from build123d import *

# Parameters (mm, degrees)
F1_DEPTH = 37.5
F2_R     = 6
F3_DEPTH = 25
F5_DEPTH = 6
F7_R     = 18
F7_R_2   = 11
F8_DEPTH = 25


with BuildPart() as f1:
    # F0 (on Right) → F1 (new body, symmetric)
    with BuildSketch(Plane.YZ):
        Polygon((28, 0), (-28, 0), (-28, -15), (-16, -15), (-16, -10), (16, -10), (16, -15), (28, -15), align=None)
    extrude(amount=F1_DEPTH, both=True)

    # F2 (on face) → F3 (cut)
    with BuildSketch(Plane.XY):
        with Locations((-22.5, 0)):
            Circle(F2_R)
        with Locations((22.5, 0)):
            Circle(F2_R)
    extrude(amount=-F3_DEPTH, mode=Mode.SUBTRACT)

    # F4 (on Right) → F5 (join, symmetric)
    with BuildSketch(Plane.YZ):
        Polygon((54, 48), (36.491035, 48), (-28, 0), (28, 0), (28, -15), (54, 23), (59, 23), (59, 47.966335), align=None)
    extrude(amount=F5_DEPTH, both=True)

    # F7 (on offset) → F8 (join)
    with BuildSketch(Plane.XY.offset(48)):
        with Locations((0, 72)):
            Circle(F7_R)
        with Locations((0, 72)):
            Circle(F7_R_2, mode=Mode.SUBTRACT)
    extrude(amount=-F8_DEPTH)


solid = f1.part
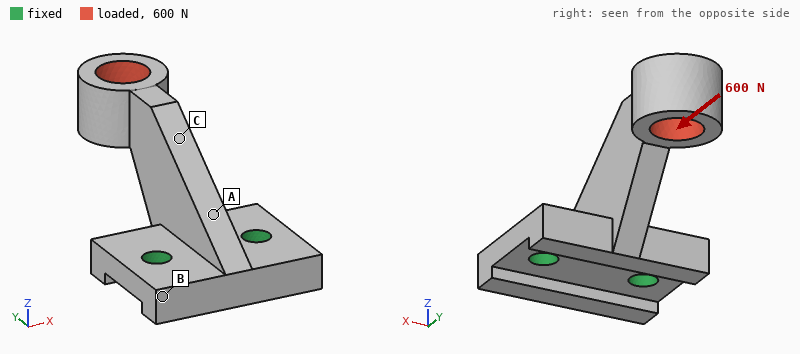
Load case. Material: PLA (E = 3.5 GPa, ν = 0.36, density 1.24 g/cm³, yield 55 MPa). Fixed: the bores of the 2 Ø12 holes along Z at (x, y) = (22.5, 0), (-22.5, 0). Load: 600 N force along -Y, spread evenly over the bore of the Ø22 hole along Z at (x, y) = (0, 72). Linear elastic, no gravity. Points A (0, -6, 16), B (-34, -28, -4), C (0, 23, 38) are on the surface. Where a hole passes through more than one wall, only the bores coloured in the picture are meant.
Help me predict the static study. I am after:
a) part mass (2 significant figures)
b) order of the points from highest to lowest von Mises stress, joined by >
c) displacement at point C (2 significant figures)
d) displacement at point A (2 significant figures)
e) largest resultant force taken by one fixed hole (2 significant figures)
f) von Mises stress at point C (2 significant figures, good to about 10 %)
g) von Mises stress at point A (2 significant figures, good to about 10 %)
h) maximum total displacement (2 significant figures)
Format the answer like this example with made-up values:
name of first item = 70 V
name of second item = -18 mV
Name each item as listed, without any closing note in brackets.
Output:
part mass = 110 g
order of the points from highest to lowest von Mises stress, joined by > = A > C > B
displacement at point C = 0.39 mm
displacement at point A = 0.15 mm
largest resultant force taken by one fixed hole = 310 N
von Mises stress at point C = 3.7 MPa
von Mises stress at point A = 6.5 MPa
maximum total displacement = 0.92 mm
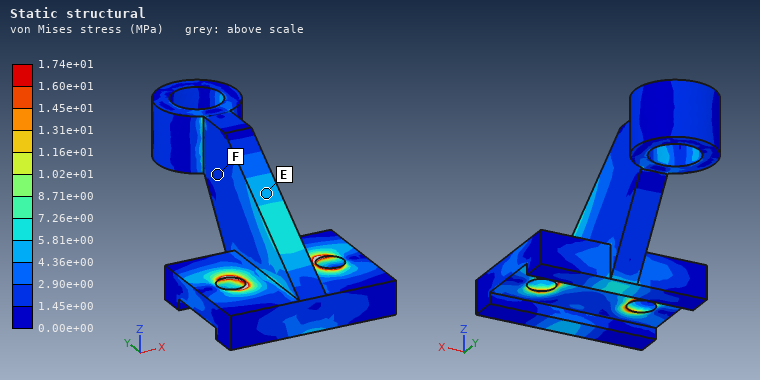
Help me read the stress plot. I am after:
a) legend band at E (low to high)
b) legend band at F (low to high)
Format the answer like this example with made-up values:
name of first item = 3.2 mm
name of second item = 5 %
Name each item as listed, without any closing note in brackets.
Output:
legend band at E = 4.36e+00 to 5.81e+00 MPa
legend band at F = 1.45e+00 to 2.90e+00 MPa
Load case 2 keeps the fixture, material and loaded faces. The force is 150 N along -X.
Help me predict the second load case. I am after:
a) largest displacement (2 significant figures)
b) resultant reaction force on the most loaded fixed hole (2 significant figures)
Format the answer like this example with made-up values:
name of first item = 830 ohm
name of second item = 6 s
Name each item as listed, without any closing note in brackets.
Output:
largest displacement = 1.4 mm
resultant reaction force on the most loaded fixed hole = 280 N
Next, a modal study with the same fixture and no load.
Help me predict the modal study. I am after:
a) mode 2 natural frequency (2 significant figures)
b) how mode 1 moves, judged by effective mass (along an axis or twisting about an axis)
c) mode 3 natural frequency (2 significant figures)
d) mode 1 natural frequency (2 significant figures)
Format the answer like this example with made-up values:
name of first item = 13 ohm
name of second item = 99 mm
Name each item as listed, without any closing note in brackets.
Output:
mode 2 natural frequency = 600 Hz
how mode 1 moves, judged by effective mass = along X
mode 3 natural frequency = 1200 Hz
mode 1 natural frequency = 410 Hz
